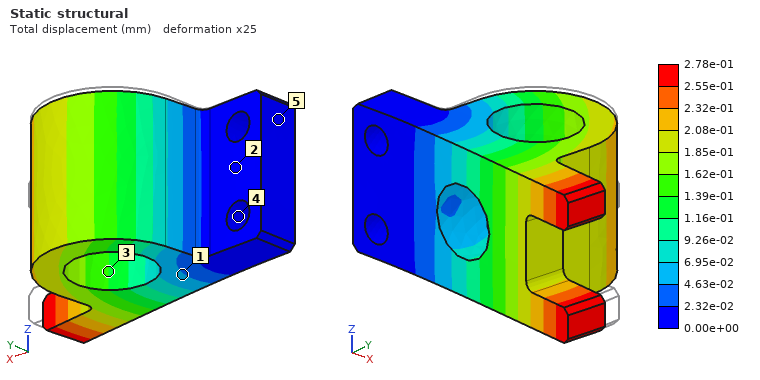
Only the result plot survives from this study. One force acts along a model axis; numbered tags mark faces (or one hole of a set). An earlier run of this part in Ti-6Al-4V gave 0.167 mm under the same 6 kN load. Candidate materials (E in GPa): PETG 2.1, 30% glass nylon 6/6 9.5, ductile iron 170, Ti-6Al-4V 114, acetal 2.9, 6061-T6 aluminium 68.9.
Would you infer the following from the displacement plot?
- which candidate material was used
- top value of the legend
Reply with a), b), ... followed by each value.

a) 6061-T6 aluminium
b) 2.78e-01 mm
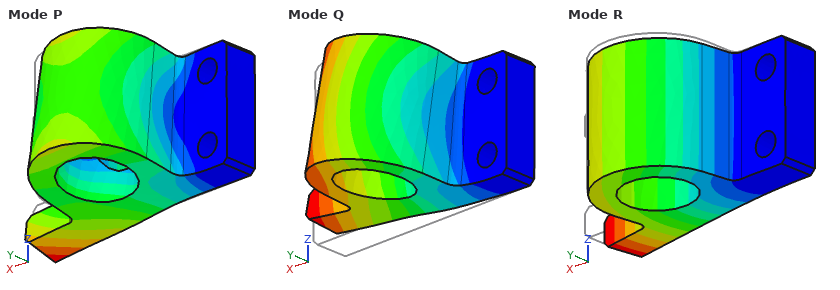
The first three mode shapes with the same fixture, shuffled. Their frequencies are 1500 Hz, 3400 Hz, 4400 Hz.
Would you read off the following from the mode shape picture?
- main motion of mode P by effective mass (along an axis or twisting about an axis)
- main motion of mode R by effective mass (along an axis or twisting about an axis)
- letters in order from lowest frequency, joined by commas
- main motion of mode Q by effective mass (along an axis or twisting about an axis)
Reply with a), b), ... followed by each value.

a) twisting about X
b) along Y
c) R, Q, P
d) along Z
